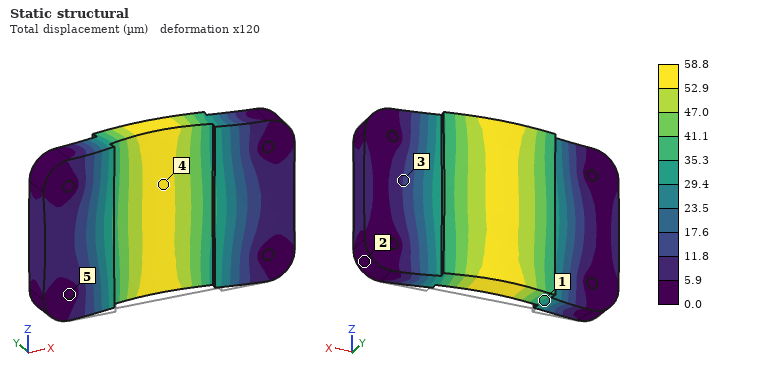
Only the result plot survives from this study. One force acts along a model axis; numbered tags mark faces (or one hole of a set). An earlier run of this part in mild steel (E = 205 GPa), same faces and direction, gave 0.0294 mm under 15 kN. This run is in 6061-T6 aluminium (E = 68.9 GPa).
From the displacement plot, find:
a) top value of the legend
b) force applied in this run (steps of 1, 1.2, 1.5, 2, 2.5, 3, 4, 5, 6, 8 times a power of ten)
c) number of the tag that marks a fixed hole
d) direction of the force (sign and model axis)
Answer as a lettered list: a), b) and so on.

a) 58.8 µm
b) 10 kN
c) 5
d) +Y
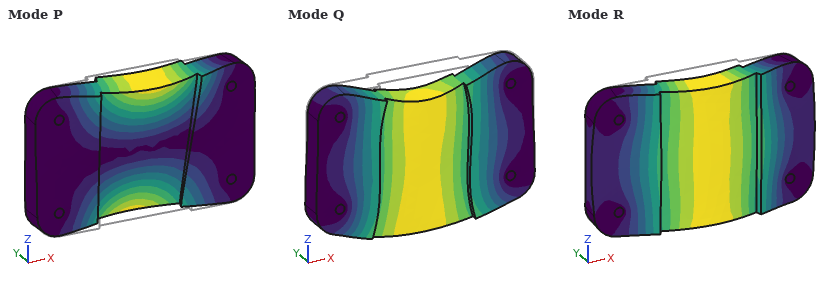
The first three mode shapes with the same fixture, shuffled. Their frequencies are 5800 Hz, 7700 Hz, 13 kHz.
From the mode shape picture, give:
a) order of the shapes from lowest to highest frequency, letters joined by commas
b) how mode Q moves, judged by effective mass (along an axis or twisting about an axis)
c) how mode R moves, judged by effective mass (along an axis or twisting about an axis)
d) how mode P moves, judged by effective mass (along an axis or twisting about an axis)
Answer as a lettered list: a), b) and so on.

a) R, P, Q
b) along Z
c) along Y
d) twisting about X
